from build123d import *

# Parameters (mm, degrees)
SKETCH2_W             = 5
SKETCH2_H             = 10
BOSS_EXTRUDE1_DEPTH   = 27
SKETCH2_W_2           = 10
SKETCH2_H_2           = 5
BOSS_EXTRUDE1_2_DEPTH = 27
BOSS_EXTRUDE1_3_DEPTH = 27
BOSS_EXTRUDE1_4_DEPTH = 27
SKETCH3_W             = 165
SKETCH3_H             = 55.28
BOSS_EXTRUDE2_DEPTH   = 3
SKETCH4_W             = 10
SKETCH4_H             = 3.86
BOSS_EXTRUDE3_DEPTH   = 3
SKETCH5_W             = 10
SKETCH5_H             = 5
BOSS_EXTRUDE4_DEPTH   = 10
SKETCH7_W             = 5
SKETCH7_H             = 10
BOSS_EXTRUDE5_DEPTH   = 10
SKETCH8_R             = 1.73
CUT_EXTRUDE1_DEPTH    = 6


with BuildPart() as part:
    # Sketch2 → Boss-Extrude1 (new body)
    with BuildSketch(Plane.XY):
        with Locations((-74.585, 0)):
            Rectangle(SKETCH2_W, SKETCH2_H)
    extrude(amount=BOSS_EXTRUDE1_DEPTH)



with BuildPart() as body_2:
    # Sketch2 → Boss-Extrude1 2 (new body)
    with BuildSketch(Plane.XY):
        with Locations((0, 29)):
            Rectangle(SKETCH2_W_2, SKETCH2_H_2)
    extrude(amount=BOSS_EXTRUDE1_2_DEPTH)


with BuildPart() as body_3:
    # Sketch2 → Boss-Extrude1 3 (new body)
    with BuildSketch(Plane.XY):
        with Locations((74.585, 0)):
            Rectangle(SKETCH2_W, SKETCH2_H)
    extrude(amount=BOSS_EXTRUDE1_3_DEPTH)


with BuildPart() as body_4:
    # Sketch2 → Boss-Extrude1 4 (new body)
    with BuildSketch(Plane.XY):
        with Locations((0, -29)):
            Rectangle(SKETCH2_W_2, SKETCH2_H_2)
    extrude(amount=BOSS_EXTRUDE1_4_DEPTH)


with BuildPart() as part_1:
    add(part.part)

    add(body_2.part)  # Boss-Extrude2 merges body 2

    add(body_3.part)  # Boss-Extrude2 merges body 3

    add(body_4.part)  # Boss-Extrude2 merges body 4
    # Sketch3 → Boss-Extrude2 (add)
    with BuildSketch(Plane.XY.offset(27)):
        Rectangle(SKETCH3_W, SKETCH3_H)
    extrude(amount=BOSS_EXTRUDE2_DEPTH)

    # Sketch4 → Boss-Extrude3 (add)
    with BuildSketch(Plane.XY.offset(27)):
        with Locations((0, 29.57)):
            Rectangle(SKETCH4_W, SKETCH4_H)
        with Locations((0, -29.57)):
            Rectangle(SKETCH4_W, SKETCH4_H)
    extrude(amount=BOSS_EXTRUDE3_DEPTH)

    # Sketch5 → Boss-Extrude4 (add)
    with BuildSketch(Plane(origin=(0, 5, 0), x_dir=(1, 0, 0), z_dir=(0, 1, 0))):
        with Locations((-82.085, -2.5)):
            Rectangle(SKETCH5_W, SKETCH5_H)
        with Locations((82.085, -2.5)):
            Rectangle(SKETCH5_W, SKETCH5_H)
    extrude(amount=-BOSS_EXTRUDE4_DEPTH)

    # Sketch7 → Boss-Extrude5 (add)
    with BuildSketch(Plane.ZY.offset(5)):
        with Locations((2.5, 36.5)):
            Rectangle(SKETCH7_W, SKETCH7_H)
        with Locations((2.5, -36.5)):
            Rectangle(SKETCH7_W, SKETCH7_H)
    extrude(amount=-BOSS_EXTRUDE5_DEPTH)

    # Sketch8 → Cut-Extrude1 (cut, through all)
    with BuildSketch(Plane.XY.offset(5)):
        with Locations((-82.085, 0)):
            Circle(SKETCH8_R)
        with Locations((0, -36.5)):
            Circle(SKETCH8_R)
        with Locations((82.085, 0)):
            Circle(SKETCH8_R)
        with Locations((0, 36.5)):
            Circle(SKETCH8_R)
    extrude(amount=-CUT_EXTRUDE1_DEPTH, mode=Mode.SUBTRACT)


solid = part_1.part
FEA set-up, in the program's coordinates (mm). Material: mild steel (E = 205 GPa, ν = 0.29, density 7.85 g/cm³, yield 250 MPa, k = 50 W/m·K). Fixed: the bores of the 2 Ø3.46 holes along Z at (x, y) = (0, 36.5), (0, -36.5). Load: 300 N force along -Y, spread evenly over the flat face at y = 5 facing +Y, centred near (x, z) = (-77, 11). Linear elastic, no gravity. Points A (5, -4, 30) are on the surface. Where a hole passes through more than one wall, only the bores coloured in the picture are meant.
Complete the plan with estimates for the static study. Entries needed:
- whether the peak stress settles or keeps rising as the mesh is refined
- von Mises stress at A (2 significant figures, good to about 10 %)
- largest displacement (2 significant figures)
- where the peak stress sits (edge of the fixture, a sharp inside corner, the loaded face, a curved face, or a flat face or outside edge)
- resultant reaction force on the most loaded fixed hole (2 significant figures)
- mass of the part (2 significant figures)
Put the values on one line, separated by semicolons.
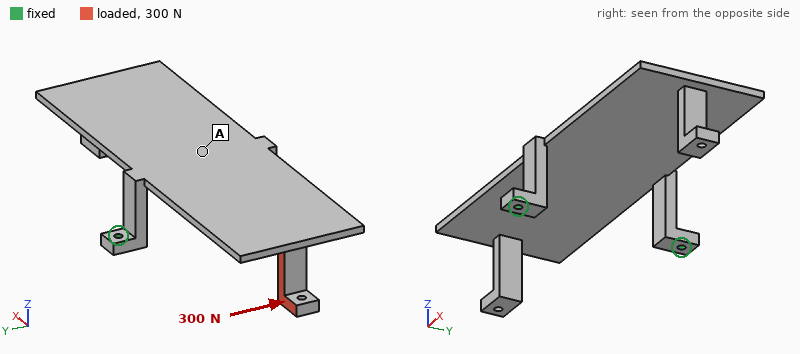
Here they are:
keeps rising; 39 MPa; 0.58 mm; edge of the fixture; 370 N; 270 g
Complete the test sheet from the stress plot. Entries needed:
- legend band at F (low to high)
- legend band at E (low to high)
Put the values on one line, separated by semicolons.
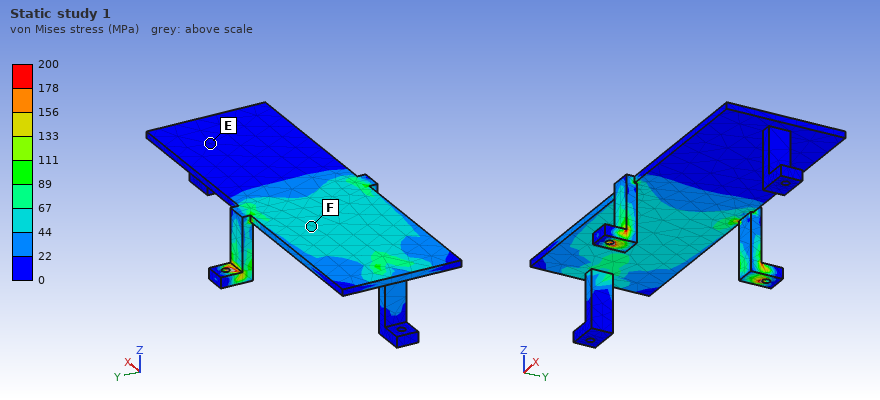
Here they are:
44 to 67 MPa; 0 to 22 MPa
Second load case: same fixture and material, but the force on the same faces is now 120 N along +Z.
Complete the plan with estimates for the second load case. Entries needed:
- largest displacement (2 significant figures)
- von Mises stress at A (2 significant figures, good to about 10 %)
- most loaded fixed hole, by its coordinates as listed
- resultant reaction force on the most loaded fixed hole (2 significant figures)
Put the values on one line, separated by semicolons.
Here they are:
1.3 mm; 30 MPa; (0, 36.5); 85 N
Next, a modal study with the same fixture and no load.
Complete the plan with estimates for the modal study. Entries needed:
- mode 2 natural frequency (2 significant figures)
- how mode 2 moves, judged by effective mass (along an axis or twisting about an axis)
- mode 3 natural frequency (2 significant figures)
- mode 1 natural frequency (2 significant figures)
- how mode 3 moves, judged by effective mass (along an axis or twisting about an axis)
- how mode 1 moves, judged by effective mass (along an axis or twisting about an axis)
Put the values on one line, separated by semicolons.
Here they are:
300 Hz; along Z; 590 Hz; 210 Hz; twisting about Z; twisting about Y
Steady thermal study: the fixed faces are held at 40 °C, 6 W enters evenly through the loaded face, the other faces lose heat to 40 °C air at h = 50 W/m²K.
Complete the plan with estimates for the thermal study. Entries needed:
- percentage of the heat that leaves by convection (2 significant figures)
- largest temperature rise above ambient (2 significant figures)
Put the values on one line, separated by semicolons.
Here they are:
97 %; 49 K
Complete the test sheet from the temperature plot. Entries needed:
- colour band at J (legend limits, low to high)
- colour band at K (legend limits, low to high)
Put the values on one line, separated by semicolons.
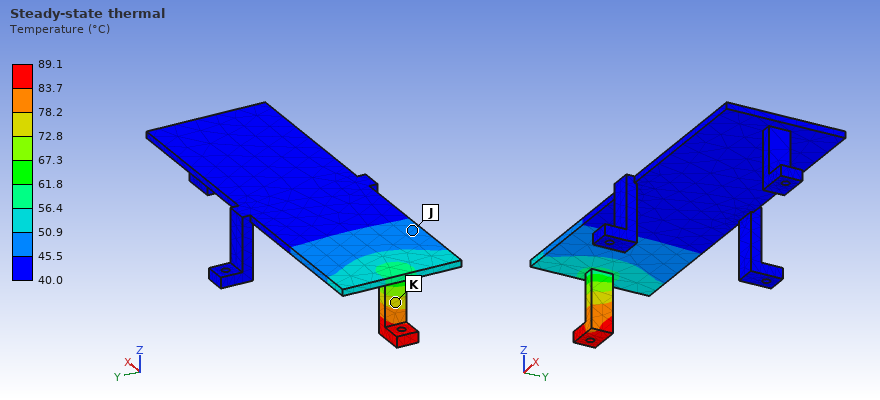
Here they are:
45.5 to 50.9 °C; 72.8 to 78.2 °C
